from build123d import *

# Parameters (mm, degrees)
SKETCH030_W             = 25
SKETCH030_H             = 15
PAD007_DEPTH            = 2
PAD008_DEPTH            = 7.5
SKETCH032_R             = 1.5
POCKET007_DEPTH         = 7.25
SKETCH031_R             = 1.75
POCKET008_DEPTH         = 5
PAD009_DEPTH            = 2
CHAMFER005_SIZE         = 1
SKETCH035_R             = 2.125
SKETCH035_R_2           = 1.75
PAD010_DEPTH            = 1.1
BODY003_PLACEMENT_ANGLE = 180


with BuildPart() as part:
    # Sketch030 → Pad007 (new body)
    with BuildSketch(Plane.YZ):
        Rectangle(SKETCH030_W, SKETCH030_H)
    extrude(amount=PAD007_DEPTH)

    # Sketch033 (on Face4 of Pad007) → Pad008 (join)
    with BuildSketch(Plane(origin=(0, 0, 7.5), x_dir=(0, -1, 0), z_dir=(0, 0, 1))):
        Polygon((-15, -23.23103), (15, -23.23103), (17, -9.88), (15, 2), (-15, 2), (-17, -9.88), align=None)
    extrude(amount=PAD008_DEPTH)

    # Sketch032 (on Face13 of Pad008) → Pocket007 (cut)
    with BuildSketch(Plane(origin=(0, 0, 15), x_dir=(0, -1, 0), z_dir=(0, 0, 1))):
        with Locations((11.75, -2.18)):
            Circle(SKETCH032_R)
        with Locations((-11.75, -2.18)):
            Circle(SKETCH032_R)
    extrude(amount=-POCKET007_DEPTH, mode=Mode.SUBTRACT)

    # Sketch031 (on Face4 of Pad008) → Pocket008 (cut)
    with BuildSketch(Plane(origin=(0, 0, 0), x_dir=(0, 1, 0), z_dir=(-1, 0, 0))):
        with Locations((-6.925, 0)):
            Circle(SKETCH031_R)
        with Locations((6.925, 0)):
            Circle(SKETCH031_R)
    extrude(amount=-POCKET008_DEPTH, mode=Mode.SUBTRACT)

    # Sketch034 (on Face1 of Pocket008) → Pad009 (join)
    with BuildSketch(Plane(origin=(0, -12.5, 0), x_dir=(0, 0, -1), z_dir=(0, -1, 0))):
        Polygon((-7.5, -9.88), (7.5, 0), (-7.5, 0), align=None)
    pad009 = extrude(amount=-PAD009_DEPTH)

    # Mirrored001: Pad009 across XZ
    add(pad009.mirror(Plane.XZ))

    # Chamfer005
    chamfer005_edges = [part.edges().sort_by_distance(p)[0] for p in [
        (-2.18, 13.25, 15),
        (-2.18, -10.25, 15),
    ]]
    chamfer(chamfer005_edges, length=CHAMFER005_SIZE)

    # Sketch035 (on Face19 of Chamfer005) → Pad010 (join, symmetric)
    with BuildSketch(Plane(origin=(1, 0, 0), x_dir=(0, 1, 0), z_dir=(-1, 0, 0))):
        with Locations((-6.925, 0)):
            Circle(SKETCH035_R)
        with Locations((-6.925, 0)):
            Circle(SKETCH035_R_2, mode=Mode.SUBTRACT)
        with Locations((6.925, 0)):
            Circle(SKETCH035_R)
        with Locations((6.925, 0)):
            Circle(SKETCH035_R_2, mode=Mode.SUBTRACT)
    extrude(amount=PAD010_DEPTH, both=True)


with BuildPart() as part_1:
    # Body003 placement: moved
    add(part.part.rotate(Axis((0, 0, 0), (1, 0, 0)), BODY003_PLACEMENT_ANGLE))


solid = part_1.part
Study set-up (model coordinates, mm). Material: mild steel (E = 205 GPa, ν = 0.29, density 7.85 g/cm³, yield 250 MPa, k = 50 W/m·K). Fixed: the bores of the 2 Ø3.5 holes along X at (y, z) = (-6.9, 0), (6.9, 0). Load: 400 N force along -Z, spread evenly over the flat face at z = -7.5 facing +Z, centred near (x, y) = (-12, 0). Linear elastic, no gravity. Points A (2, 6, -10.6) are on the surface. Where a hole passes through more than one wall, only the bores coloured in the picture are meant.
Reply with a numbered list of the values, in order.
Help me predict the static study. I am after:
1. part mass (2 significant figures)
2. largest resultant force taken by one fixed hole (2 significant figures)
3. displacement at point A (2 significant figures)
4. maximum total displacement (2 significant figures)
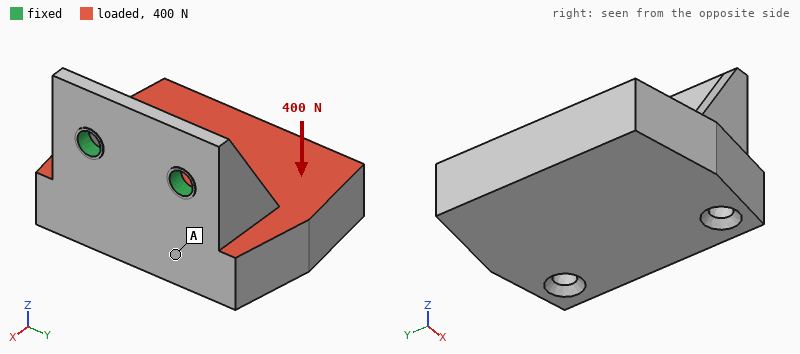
1. 55 g
2. 200 N
3. 19 µm
4. 62 µm
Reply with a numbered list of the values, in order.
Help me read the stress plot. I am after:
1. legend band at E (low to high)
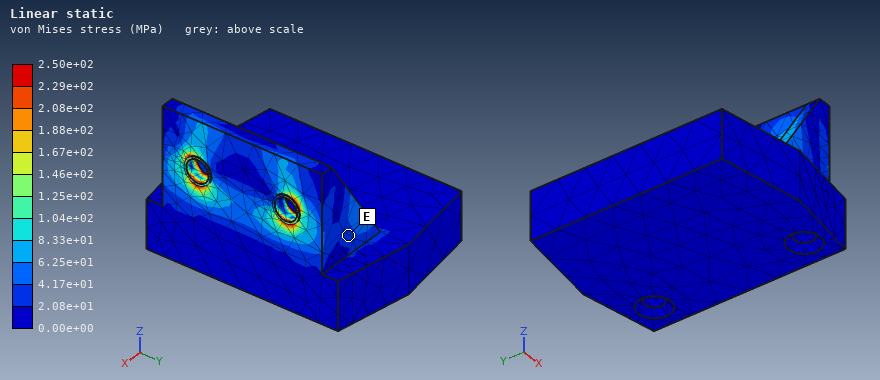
1. 2.08e+01 to 4.17e+01 MPa
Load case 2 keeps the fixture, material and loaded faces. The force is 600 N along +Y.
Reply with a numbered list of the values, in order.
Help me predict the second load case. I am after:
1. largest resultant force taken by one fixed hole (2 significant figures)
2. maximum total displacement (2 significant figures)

1. 550 N
2. 25 µm
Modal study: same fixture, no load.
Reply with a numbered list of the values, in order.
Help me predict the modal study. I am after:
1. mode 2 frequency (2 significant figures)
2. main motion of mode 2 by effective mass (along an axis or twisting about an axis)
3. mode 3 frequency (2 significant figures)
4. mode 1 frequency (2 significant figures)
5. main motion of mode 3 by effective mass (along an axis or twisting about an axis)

1. 4400 Hz
2. along Y
3. 11 kHz
4. 2100 Hz
5. along X
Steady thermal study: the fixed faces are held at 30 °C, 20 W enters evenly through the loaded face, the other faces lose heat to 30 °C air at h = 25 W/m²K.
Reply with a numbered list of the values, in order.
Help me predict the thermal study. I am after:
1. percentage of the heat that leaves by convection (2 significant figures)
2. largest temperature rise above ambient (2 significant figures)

1. 15 %
2. 64 K
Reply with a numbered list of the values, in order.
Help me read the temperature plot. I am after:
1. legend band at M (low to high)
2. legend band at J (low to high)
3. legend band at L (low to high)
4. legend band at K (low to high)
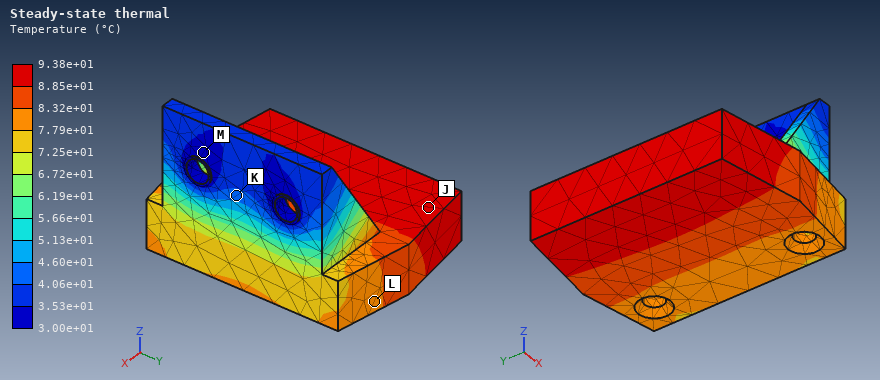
1. 3.00e+01 to 3.53e+01 °C
2. 8.85e+01 to 9.38e+01 °C
3. 7.79e+01 to 8.32e+01 °C
4. 4.06e+01 to 4.60e+01 °C
